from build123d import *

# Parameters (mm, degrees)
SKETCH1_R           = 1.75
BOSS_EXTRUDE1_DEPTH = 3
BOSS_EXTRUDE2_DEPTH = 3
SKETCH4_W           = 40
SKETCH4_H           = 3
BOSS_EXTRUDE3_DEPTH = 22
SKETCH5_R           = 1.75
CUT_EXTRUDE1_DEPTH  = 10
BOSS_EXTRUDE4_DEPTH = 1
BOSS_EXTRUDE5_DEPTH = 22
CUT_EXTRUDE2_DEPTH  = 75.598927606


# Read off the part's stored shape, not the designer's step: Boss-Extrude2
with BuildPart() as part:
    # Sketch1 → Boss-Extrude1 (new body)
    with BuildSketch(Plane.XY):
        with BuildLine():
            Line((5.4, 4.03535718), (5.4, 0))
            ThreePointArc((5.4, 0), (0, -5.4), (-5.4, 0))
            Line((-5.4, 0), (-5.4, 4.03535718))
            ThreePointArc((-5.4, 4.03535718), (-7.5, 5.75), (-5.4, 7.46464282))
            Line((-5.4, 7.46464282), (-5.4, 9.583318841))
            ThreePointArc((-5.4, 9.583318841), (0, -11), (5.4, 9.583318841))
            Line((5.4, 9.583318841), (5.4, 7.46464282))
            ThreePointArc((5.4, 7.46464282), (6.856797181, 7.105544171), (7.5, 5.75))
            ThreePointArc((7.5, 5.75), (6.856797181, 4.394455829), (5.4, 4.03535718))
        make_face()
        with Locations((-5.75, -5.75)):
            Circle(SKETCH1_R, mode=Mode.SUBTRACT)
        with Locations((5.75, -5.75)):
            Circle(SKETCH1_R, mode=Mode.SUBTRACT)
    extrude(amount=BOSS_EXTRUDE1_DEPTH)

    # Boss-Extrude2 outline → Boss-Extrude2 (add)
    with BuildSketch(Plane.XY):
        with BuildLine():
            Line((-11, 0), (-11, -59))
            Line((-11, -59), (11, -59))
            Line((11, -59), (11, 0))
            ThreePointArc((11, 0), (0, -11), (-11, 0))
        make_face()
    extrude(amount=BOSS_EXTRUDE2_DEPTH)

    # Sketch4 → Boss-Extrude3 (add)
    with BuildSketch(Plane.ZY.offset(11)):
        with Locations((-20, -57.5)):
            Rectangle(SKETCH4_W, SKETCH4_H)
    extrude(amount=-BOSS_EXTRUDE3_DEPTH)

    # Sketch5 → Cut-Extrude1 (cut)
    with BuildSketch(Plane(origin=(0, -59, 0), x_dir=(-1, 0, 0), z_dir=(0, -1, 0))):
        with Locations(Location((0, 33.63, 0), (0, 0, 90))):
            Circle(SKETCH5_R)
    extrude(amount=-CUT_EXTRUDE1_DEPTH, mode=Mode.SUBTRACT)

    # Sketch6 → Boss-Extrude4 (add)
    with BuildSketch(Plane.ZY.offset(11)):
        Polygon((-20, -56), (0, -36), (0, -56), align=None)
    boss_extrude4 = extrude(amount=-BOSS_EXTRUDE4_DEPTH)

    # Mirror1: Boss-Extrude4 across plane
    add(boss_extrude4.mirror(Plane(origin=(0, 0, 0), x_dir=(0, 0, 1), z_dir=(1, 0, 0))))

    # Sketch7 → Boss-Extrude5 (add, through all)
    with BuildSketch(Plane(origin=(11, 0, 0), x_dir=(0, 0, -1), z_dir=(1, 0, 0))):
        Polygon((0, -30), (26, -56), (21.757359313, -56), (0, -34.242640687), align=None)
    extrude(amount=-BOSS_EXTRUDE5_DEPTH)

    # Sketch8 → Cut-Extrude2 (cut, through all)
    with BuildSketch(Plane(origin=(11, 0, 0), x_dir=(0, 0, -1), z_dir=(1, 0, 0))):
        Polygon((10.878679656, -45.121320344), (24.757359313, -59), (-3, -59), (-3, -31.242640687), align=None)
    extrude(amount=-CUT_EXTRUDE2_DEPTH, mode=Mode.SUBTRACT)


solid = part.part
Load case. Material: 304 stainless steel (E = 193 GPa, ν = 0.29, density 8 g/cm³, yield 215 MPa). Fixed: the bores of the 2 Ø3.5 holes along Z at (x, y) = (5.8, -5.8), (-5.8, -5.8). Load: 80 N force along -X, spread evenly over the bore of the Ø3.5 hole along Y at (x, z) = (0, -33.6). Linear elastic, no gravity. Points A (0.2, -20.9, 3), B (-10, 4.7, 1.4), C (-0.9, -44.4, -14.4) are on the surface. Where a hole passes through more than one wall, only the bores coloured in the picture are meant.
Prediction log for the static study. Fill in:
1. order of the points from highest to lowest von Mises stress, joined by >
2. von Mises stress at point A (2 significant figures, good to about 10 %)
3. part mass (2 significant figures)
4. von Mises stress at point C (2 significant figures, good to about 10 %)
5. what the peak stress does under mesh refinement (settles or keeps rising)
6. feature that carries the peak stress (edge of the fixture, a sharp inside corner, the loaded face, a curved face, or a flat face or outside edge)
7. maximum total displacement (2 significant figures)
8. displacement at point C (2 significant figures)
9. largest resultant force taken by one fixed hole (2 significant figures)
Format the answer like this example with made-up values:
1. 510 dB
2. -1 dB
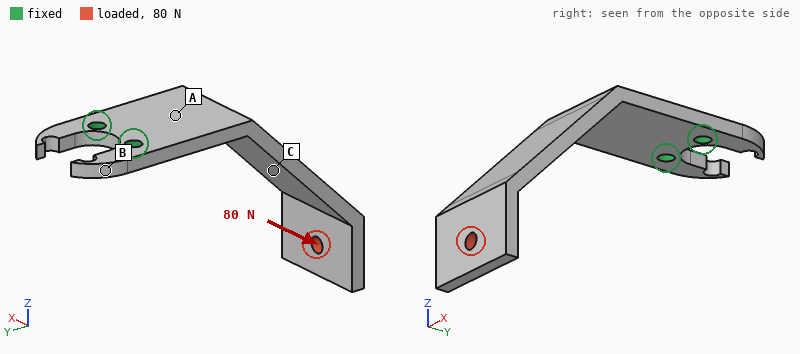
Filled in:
1. A > C > B
2. 67 MPa
3. 44 g
4. 17 MPa
5. keeps rising
6. edge of the fixture
7. 0.19 mm
8. 0.065 mm
9. 350 N
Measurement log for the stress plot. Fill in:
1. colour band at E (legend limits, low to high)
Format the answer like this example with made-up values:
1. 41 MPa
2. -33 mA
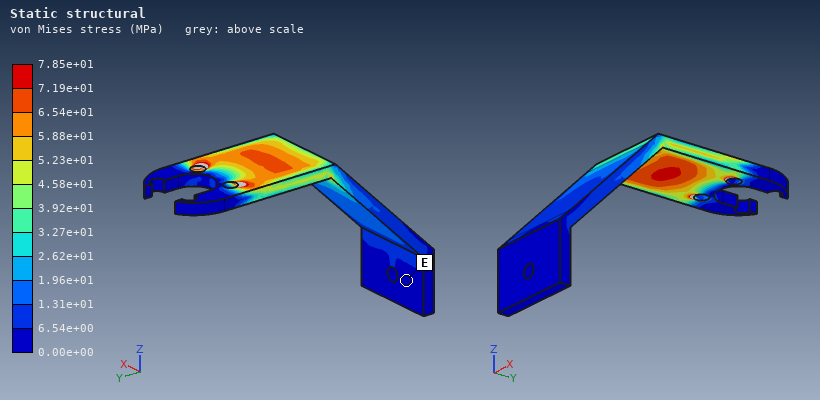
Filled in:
1. 0.00e+00 to 6.54e+00 MPa
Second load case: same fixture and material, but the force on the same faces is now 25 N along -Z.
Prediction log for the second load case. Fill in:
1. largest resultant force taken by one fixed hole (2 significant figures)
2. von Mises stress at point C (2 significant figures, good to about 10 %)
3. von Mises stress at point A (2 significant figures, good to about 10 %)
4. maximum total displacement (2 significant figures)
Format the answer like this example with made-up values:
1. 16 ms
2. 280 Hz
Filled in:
1. 13 N
2. 8.7 MPa
3. 25 MPa
4. 0.19 mm
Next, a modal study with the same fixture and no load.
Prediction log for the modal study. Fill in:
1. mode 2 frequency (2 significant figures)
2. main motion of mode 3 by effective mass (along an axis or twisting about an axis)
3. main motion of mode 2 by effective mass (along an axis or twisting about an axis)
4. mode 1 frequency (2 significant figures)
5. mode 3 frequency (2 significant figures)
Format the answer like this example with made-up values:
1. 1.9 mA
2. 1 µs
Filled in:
1. 1100 Hz
2. along Z
3. along X
4. 450 Hz
5. 2100 Hz
